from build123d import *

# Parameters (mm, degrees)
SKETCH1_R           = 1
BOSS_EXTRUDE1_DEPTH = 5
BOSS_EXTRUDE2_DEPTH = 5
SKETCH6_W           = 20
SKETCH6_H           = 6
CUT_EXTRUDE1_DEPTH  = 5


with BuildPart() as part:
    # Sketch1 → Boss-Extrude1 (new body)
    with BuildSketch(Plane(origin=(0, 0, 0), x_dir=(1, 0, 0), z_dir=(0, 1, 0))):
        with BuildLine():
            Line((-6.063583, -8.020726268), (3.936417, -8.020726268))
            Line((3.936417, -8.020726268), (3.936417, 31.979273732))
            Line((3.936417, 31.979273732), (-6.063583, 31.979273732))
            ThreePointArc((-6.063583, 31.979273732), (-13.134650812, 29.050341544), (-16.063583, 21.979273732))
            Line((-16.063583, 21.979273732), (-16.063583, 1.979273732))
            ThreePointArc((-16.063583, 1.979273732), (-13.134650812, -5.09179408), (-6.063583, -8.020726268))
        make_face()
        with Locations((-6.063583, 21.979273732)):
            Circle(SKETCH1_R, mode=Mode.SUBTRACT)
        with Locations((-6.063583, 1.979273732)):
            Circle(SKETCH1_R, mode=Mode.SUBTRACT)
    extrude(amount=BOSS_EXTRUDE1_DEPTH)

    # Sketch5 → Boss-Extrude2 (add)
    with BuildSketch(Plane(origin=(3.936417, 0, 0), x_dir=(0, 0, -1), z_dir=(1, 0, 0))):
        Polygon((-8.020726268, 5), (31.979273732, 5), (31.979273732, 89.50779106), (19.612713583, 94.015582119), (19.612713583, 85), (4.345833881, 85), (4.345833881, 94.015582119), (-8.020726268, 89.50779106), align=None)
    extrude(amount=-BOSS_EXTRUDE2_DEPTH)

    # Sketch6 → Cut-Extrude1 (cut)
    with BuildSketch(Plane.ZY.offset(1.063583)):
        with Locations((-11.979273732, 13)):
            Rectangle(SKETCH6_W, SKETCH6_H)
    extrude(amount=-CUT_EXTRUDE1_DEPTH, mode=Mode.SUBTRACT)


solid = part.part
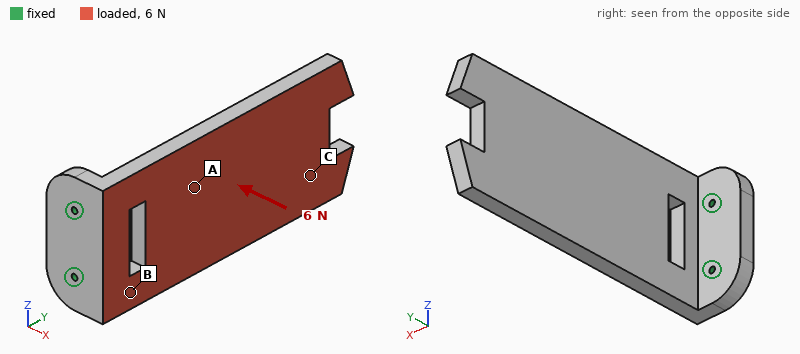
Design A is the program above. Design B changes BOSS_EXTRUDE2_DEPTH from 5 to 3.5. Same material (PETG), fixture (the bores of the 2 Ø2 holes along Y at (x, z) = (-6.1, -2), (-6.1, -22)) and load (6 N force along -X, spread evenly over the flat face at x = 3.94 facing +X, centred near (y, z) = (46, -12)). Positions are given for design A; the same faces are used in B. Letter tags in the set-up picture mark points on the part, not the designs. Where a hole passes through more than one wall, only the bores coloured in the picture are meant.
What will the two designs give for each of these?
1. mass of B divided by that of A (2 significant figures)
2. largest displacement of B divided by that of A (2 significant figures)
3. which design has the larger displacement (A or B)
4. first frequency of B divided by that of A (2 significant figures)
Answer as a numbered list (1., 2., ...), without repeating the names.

1. 0.76
2. 2.4
3. B
4. 0.77
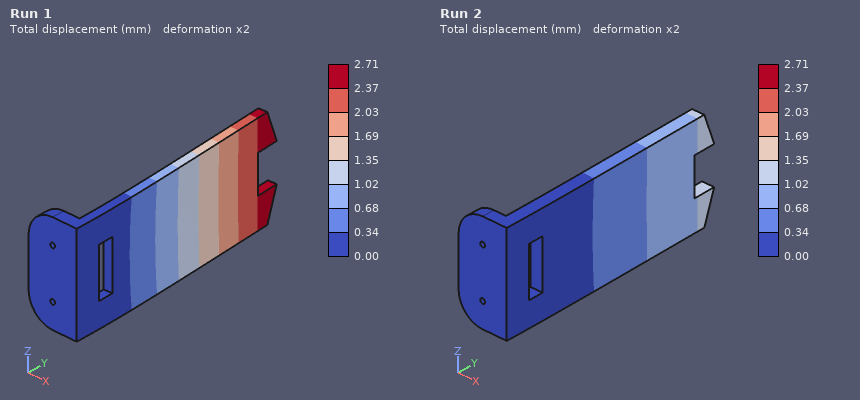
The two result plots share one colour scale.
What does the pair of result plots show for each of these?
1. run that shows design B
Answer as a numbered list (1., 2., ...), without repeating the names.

1. Run 1
